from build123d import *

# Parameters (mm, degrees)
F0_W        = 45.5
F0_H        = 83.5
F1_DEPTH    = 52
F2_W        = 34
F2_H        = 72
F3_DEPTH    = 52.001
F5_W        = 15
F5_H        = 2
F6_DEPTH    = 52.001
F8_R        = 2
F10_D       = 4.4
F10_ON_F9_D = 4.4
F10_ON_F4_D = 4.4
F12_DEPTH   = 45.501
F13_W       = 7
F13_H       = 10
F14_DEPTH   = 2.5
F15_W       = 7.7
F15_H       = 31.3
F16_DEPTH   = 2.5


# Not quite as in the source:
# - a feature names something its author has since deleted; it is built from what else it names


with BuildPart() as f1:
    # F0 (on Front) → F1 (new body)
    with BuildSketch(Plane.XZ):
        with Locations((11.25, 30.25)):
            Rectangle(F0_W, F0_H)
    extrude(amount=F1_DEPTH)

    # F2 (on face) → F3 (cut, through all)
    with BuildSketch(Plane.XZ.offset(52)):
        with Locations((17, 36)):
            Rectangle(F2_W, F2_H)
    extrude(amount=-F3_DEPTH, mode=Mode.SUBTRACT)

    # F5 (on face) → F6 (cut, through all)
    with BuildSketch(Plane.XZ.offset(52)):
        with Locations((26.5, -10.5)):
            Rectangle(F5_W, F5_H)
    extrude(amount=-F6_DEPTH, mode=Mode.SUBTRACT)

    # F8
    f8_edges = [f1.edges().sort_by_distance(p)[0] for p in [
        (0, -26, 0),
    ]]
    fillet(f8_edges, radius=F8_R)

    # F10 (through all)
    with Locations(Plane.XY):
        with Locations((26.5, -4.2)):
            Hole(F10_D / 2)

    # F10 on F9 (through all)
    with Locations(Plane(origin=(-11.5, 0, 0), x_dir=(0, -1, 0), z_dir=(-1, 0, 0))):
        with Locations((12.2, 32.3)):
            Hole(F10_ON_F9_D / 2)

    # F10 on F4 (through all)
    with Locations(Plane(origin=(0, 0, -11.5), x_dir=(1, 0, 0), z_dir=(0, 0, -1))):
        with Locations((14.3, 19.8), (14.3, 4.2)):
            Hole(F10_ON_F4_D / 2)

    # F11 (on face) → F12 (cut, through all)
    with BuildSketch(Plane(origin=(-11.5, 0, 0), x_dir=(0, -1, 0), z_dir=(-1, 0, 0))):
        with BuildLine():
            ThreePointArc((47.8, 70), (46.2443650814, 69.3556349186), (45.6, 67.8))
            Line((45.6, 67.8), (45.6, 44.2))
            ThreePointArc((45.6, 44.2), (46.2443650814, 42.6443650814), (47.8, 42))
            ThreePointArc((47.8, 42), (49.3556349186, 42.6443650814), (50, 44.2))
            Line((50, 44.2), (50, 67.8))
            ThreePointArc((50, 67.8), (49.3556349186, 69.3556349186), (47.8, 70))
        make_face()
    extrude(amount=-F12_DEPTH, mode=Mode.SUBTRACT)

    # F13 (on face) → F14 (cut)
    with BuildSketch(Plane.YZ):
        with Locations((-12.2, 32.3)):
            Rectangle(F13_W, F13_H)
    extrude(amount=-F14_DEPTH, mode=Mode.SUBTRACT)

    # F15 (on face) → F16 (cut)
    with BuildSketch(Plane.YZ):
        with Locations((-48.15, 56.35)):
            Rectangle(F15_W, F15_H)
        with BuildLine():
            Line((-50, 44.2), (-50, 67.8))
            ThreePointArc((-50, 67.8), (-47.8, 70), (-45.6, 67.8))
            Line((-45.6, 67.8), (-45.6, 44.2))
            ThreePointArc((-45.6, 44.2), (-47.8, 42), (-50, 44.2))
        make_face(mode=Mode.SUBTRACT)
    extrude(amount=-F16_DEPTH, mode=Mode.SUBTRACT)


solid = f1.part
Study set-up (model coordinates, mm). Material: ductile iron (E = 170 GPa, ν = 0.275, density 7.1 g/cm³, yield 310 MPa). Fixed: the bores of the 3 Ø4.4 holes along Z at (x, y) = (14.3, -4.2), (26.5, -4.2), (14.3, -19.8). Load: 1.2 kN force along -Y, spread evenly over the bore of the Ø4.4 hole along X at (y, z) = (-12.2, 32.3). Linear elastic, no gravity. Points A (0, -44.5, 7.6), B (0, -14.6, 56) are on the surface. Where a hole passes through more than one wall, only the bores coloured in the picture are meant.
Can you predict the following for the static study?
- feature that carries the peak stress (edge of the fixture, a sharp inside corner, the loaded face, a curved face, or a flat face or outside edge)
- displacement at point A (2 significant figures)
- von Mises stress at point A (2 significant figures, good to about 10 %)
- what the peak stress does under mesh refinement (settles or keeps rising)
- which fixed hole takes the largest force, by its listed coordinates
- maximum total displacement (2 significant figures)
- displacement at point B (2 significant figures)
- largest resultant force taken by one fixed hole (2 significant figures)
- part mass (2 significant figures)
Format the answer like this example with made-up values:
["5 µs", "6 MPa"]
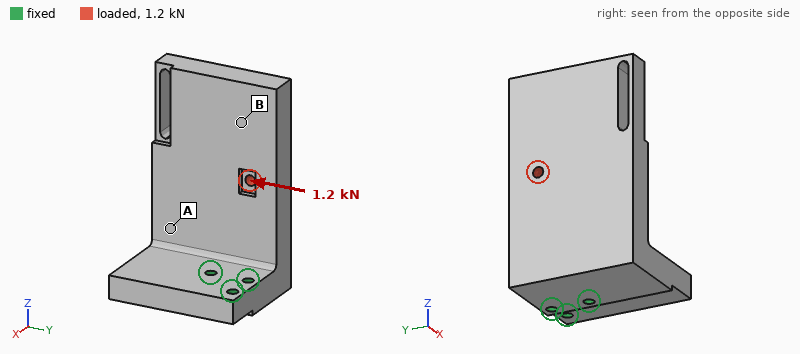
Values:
["edge of the fixture", "17 µm", "9.2 MPa", "keeps rising", "(14.3, -19.8)", "49 µm", "36 µm", "2.3 kN", "470 g"]
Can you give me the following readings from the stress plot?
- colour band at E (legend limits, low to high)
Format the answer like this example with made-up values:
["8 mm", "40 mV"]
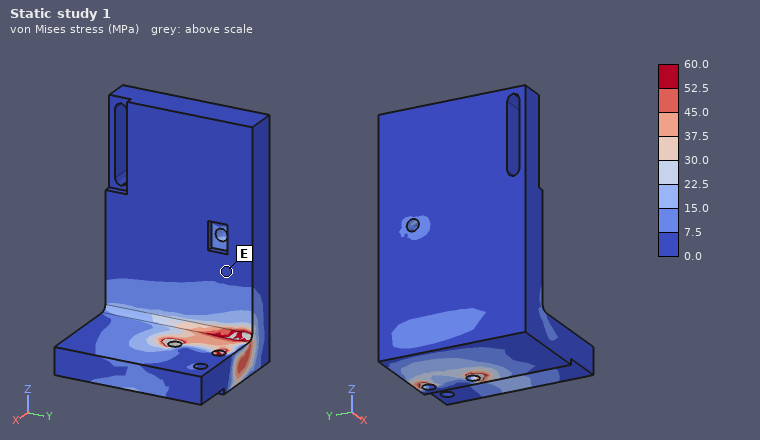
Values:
["0.0 to 7.5 MPa"]
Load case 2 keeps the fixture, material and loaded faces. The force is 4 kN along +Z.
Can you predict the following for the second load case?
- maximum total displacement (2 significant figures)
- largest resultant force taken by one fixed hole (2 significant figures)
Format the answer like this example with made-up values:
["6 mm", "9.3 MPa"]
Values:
["0.11 mm", "2.3 kN"]
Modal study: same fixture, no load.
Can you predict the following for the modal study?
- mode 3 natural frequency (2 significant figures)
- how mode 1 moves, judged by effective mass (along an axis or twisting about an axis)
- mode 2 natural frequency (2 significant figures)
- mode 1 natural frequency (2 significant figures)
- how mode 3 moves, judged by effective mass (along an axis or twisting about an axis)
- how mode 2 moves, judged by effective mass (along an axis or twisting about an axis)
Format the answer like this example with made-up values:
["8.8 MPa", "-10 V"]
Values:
["4300 Hz", "along X", "1700 Hz", "1000 Hz", "twisting about Z", "along Y"]
